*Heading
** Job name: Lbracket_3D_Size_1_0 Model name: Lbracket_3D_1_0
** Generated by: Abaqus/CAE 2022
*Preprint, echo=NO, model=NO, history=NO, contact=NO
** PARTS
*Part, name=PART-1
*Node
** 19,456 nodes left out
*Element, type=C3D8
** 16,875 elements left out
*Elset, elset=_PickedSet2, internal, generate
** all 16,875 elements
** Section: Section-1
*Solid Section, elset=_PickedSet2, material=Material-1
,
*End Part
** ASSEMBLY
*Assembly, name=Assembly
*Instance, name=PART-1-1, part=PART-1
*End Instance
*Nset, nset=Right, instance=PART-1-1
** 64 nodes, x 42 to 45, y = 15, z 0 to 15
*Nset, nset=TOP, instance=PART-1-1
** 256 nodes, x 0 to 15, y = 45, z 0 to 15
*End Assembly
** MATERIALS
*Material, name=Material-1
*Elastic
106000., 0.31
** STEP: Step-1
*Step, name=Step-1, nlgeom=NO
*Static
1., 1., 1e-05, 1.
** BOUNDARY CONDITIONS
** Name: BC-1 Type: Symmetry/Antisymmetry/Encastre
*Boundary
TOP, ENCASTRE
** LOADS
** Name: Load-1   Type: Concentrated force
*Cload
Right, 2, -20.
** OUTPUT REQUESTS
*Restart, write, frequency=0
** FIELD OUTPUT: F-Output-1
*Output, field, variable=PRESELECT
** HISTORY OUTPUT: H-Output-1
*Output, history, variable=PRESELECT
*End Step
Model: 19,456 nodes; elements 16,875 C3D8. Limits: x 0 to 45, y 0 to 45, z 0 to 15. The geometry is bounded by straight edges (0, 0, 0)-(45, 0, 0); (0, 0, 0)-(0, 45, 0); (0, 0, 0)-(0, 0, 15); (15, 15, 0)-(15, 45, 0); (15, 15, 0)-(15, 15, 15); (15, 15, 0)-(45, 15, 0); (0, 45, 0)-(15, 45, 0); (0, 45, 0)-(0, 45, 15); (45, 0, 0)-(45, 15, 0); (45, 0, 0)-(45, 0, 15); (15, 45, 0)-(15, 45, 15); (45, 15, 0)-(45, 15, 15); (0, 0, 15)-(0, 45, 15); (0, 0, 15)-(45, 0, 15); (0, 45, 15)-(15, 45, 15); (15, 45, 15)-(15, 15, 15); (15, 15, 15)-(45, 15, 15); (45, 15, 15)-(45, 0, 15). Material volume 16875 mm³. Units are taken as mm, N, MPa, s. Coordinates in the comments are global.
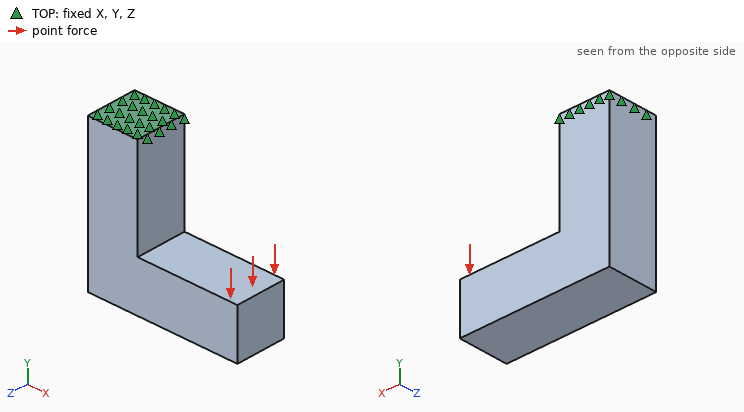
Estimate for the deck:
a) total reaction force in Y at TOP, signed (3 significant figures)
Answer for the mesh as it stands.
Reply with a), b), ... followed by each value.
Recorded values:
a) 1280 N
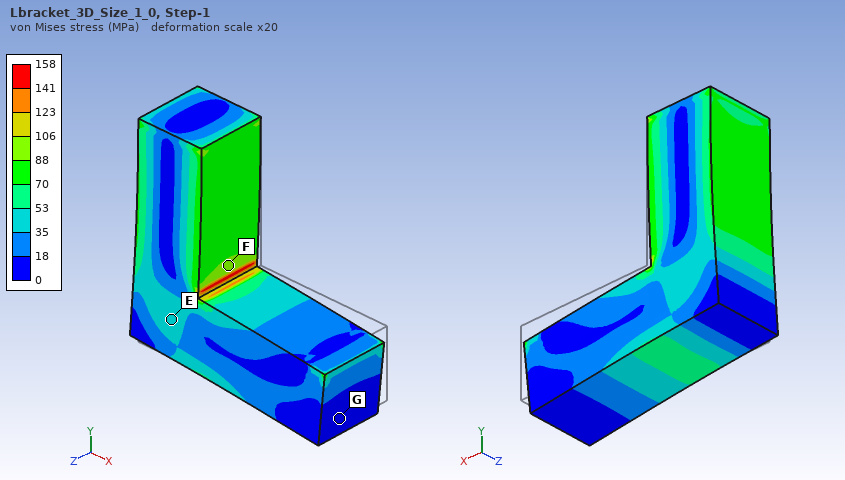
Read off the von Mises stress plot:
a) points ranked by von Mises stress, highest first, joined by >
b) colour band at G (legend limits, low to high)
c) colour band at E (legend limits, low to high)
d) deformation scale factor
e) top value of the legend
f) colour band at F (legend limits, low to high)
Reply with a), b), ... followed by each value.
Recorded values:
a) F > E > G
b) 0 to 18 MPa
c) 35 to 53 MPa
d) 20
e) 158 MPa
f) 88 to 106 MPa
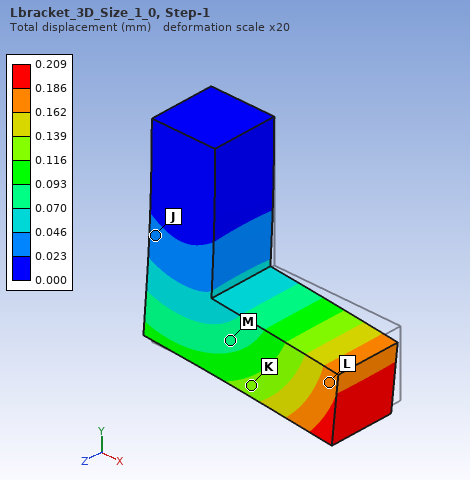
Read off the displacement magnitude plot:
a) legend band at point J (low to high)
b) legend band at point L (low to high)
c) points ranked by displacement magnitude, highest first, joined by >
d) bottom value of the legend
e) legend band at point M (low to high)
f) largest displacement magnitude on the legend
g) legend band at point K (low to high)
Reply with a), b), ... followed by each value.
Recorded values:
a) 0.023 to 0.046 mm
b) 0.162 to 0.186 mm
c) L > K > M > J
d) 0.000 mm
e) 0.070 to 0.093 mm
f) 0.209 mm
g) 0.116 to 0.139 mm
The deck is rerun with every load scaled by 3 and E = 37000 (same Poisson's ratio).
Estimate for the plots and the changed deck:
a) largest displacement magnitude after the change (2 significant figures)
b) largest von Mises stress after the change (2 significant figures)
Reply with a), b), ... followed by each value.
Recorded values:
a) 1.8 mm
b) 470 MPa
